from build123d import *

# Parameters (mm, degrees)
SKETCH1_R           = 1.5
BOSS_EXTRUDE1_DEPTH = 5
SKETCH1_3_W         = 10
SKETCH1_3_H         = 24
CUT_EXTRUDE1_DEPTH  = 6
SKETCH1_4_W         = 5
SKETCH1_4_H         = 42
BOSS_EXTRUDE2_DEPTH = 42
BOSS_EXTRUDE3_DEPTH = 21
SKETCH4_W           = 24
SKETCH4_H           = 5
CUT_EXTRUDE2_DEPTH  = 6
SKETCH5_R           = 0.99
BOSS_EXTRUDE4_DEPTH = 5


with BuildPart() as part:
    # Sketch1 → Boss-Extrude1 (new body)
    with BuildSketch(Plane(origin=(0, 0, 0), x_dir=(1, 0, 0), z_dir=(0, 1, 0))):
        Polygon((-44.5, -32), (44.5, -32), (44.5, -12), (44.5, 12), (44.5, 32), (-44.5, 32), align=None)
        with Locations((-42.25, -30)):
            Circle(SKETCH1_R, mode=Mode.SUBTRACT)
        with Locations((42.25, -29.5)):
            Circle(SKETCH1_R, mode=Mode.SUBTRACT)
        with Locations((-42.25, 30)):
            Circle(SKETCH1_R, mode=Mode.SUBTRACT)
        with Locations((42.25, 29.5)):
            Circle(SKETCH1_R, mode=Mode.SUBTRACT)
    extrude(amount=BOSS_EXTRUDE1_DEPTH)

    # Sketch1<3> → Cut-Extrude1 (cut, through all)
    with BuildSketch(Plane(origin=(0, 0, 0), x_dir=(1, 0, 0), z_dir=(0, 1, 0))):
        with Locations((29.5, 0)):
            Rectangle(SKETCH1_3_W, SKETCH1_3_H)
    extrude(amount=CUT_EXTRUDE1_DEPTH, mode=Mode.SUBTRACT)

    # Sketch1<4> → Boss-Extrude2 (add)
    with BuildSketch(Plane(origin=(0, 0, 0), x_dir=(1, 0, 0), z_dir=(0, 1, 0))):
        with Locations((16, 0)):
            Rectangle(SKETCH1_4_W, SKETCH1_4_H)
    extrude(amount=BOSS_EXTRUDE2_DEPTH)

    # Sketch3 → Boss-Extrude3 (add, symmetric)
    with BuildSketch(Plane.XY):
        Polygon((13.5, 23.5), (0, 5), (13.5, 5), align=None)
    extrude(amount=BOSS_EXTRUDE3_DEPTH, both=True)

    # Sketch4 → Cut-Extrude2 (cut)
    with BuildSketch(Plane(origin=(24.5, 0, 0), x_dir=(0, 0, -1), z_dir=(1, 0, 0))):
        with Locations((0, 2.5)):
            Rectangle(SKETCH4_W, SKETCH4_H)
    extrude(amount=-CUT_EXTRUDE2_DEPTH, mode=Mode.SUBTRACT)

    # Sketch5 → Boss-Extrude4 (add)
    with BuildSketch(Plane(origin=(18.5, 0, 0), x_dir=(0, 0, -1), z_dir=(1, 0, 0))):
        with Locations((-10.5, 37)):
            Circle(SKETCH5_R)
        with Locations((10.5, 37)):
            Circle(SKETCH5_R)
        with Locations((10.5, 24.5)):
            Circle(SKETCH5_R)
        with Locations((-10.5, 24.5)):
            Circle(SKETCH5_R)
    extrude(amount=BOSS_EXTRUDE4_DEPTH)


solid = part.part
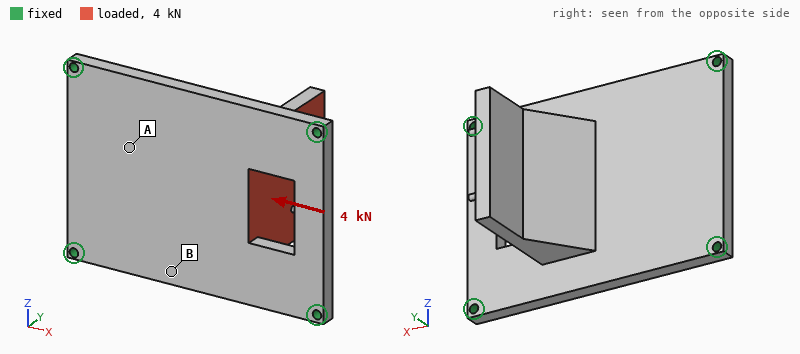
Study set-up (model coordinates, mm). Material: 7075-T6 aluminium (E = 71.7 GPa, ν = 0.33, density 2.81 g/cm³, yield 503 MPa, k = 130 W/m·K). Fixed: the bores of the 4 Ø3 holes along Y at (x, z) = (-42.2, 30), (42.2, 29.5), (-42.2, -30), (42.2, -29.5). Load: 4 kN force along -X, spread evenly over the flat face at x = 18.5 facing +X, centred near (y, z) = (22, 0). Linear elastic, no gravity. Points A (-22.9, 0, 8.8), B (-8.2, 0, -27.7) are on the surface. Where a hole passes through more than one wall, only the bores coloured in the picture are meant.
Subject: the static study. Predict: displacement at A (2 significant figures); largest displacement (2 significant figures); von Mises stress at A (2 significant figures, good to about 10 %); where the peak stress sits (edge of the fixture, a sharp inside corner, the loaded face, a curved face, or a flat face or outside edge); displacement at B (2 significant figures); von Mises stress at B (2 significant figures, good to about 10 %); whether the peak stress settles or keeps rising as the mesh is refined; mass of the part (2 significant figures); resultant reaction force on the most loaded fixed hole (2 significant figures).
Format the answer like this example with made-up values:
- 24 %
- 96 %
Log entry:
- 0.12 mm
- 0.45 mm
- 33 MPa
- edge of the fixture
- 0.13 mm
- 83 MPa
- keeps rising
- 110 g
- 1.3 kN
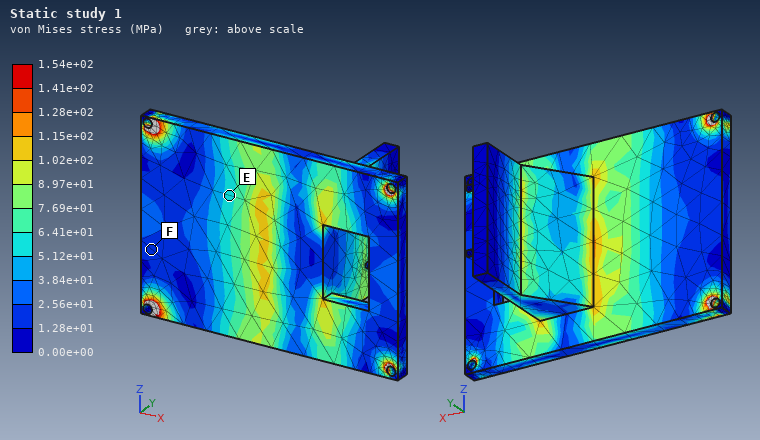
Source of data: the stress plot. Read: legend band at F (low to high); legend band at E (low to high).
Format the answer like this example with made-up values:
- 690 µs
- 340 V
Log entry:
- 1.28e+01 to 2.56e+01 MPa
- 5.12e+01 to 6.41e+01 MPa
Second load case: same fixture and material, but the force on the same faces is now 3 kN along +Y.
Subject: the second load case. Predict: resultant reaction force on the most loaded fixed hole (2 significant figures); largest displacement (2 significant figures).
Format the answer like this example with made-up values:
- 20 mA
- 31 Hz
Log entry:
- 1.2 kN
- 0.25 mm
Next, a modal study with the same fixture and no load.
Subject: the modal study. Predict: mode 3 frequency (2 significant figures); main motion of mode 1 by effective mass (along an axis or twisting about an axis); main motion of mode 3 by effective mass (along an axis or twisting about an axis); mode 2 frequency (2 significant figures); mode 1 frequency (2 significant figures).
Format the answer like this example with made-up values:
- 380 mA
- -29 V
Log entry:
- 3400 Hz
- along Y
- along X
- 2900 Hz
- 2000 Hz
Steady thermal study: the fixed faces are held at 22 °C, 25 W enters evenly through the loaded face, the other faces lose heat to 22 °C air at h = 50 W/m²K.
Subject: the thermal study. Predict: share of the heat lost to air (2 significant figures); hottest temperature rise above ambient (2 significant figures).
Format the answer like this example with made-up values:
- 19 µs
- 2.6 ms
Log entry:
- 30 %
- 24 K
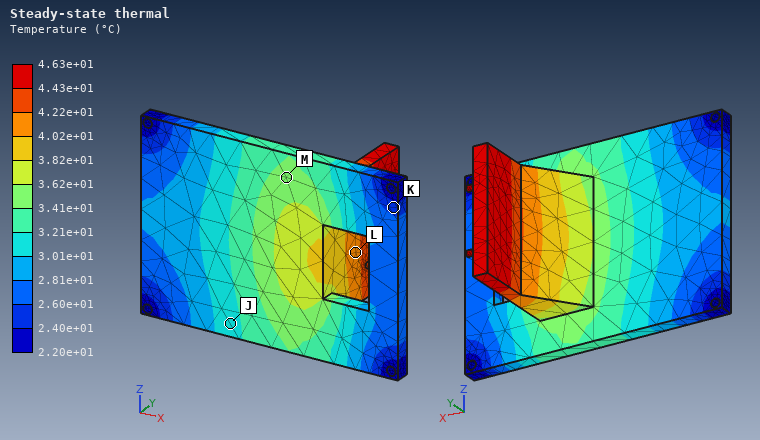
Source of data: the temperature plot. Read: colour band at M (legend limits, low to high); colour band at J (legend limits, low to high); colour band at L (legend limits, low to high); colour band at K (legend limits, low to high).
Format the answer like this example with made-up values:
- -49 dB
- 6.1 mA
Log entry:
- 3.41e+01 to 3.62e+01 °C
- 3.01e+01 to 3.21e+01 °C
- 4.02e+01 to 4.22e+01 °C
- 2.40e+01 to 2.60e+01 °C
